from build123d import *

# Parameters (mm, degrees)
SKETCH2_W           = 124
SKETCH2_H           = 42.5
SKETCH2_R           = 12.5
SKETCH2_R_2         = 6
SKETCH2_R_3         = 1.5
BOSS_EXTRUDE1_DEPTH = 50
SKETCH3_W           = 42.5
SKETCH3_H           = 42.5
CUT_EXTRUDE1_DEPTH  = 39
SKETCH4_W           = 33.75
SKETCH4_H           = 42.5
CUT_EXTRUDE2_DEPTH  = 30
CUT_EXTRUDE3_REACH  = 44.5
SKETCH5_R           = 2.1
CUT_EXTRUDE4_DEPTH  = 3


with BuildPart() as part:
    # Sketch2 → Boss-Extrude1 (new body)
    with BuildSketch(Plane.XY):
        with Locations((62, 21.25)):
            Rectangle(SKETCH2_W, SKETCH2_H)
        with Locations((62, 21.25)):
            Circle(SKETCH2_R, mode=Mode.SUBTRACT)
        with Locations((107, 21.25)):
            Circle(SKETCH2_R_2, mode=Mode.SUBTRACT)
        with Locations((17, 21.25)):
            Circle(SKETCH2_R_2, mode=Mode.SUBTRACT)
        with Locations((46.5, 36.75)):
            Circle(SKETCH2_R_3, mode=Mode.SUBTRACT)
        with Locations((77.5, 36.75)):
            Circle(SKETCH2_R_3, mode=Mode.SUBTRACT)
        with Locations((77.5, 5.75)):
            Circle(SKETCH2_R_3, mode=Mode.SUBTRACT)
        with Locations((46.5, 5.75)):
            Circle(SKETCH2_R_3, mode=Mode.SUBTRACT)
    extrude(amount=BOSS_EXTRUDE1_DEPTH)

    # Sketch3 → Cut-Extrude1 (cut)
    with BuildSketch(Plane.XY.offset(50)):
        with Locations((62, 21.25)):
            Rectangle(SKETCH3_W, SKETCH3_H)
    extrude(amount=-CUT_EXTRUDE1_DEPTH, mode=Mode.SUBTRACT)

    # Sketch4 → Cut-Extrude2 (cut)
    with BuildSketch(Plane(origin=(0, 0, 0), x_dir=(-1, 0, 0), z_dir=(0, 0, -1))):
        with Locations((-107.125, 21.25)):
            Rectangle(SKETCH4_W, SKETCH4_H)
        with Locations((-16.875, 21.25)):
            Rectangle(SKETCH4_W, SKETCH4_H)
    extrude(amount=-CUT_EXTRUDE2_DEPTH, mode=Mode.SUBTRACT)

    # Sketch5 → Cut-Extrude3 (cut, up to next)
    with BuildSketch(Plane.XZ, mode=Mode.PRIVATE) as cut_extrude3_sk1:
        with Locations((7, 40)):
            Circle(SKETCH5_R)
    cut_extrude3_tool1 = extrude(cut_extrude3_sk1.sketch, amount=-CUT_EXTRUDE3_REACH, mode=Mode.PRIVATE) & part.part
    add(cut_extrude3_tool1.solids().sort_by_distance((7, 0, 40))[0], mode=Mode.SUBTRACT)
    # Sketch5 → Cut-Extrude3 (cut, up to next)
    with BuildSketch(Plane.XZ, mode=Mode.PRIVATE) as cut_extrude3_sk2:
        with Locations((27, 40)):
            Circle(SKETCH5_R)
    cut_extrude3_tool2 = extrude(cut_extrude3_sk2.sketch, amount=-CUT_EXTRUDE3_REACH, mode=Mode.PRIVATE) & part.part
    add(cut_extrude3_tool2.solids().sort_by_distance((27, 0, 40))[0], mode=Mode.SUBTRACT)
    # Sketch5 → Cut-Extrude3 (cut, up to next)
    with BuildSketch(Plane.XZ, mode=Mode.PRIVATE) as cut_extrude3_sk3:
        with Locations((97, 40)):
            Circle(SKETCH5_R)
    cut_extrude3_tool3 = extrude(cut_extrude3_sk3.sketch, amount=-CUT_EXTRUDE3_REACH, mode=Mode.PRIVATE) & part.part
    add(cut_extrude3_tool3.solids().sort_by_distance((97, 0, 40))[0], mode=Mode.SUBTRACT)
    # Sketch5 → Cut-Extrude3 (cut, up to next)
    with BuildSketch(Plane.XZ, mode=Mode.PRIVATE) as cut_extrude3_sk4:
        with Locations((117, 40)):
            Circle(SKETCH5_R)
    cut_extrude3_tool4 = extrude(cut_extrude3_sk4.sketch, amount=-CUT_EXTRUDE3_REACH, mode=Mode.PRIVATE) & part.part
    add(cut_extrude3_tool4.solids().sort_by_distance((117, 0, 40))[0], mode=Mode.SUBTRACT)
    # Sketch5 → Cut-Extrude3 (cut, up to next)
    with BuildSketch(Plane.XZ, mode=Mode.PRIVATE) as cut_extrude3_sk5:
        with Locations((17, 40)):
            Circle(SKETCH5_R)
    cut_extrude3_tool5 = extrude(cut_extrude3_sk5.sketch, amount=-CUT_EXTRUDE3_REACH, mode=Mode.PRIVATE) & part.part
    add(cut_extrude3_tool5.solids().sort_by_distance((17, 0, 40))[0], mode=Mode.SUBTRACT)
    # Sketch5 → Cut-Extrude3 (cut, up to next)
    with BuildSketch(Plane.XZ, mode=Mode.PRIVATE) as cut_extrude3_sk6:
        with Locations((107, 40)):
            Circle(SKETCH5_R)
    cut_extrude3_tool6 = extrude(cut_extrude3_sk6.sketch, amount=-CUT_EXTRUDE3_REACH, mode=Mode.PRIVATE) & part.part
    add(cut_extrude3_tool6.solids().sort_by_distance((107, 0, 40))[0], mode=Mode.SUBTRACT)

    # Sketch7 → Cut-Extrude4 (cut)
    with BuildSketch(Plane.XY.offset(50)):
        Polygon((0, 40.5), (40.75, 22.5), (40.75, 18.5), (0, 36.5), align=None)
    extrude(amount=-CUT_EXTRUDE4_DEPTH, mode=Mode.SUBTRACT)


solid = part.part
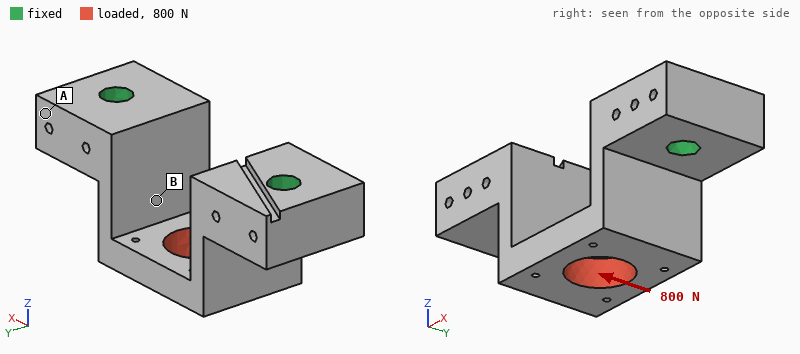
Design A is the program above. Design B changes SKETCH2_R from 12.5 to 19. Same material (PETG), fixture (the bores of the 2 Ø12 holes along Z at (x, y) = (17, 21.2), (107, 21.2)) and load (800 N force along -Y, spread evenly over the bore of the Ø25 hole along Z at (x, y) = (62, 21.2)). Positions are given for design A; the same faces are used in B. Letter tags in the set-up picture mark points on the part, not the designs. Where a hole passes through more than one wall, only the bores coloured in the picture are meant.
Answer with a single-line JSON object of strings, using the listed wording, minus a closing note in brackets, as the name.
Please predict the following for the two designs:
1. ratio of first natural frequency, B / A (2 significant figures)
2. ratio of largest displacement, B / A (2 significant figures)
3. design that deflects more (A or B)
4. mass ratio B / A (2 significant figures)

{"ratio of first natural frequency, B / A": "1.0", "ratio of largest displacement, B / A": "1.3", "design that deflects more": "B", "mass ratio B / A": "0.92"}
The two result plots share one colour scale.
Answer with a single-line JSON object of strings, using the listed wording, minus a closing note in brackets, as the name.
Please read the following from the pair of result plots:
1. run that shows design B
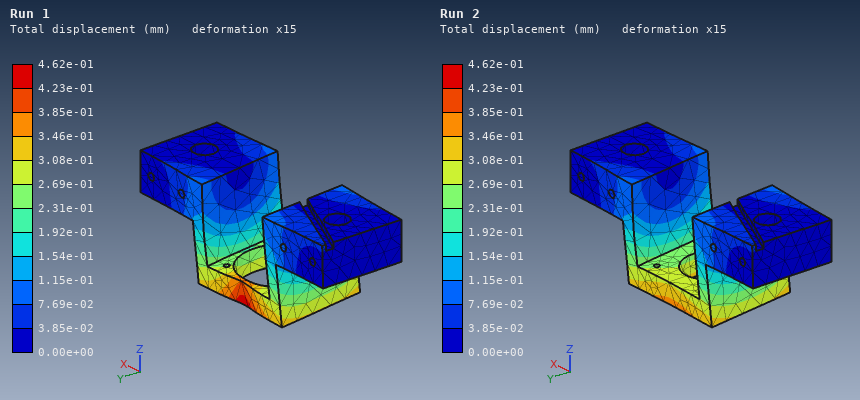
{"run that shows design B": "Run 1"}
